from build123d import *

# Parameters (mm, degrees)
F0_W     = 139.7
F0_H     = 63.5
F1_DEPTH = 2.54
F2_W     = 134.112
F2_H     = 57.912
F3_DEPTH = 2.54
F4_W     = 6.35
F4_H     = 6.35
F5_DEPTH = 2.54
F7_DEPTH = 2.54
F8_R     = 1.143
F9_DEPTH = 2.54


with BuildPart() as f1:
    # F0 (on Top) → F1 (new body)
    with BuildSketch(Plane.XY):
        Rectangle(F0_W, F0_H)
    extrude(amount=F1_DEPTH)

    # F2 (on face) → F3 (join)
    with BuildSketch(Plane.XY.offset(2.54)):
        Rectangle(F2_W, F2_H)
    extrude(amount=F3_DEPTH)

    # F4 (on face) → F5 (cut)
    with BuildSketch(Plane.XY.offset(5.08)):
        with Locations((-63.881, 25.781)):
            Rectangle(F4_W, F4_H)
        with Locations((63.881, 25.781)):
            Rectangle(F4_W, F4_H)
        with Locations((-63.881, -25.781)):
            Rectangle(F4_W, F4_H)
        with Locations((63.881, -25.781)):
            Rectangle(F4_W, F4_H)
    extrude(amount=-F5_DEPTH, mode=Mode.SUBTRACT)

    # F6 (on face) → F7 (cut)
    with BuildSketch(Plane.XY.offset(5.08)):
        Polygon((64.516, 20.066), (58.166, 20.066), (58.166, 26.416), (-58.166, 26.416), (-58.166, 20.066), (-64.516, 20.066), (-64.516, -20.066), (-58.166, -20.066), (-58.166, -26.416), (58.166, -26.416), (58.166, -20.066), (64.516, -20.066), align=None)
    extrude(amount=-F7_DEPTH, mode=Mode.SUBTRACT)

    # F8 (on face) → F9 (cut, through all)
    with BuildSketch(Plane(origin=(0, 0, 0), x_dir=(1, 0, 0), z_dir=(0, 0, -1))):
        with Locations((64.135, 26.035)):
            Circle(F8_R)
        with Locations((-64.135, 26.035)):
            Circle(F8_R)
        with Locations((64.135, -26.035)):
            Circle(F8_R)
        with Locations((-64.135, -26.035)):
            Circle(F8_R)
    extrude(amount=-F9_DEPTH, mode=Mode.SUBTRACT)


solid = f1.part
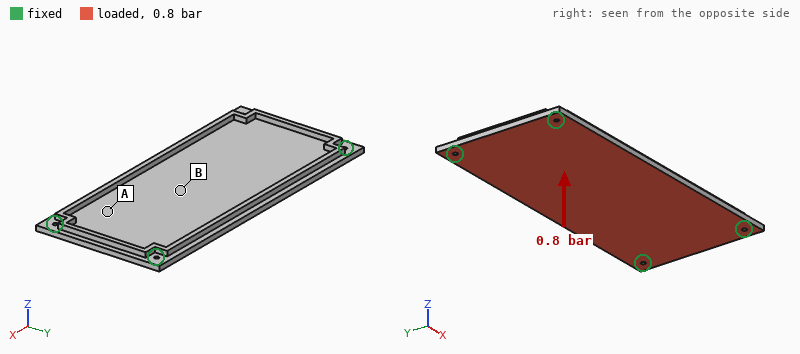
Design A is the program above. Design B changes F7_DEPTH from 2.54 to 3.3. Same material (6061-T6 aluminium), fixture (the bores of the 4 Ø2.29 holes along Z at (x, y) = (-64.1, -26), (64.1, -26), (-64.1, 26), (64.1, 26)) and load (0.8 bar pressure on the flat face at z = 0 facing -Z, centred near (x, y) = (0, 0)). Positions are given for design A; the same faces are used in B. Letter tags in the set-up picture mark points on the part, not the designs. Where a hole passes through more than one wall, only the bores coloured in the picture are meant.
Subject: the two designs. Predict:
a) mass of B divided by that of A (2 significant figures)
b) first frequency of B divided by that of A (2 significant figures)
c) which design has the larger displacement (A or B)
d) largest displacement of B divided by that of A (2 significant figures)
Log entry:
0.80
1.0
B
1.4
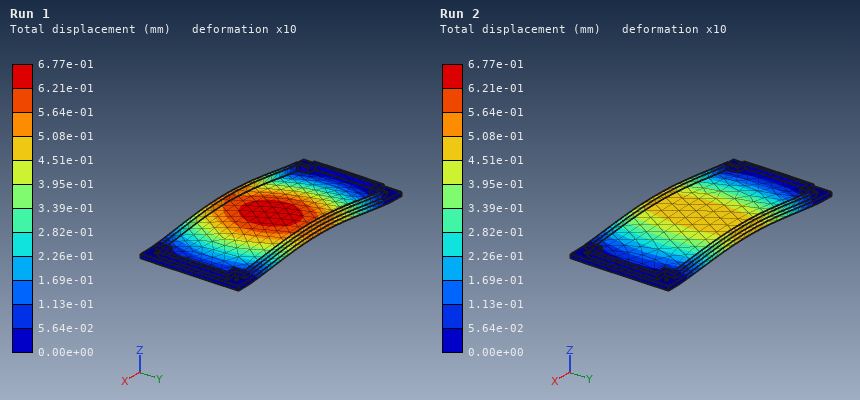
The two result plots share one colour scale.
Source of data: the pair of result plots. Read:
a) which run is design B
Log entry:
Run 1
